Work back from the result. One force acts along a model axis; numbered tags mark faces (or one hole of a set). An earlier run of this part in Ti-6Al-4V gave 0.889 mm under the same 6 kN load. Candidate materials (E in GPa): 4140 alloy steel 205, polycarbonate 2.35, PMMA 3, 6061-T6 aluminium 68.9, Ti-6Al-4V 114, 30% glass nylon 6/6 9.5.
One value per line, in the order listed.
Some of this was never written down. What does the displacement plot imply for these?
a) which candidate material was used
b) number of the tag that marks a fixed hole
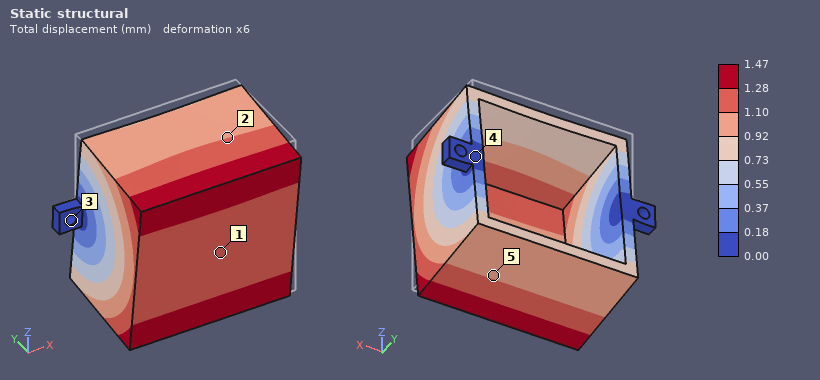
6061-T6 aluminium
3
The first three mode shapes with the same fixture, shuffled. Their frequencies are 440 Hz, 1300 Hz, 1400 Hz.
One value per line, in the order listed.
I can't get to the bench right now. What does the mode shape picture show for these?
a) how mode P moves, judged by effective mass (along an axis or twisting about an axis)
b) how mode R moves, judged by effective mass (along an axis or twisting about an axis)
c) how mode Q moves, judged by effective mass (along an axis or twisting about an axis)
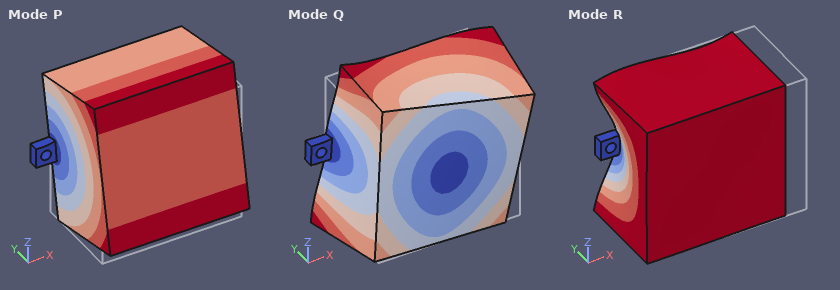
along Z
along X
twisting about Y
